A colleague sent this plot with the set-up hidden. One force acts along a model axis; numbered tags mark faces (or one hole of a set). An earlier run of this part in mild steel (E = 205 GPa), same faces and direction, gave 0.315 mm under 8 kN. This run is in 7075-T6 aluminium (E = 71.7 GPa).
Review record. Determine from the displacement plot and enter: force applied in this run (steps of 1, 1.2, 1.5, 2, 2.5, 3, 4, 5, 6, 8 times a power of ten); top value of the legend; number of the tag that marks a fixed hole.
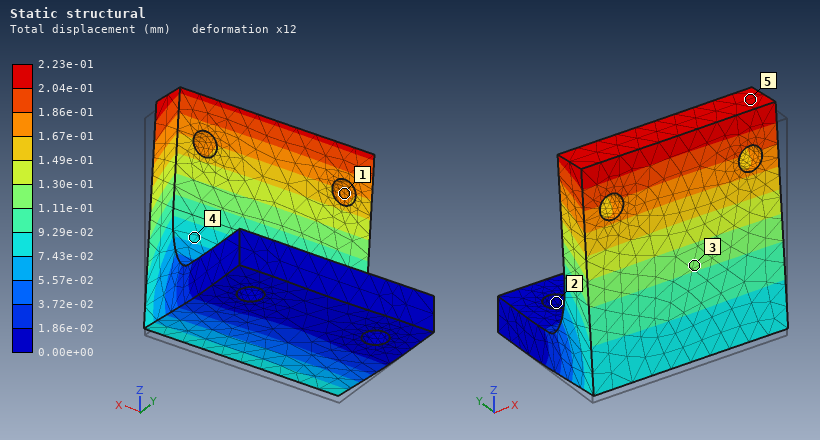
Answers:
2 kN
2.23e-01 mm
2
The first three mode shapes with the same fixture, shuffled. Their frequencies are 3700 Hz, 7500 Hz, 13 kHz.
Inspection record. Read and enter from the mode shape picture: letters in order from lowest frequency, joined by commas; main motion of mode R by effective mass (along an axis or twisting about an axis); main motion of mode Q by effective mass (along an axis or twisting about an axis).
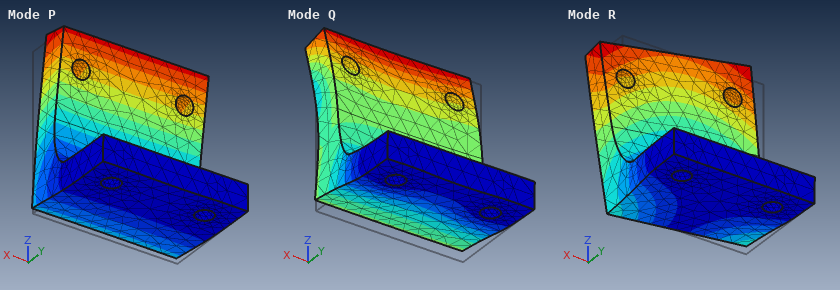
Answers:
P, R, Q
along X
along Z
